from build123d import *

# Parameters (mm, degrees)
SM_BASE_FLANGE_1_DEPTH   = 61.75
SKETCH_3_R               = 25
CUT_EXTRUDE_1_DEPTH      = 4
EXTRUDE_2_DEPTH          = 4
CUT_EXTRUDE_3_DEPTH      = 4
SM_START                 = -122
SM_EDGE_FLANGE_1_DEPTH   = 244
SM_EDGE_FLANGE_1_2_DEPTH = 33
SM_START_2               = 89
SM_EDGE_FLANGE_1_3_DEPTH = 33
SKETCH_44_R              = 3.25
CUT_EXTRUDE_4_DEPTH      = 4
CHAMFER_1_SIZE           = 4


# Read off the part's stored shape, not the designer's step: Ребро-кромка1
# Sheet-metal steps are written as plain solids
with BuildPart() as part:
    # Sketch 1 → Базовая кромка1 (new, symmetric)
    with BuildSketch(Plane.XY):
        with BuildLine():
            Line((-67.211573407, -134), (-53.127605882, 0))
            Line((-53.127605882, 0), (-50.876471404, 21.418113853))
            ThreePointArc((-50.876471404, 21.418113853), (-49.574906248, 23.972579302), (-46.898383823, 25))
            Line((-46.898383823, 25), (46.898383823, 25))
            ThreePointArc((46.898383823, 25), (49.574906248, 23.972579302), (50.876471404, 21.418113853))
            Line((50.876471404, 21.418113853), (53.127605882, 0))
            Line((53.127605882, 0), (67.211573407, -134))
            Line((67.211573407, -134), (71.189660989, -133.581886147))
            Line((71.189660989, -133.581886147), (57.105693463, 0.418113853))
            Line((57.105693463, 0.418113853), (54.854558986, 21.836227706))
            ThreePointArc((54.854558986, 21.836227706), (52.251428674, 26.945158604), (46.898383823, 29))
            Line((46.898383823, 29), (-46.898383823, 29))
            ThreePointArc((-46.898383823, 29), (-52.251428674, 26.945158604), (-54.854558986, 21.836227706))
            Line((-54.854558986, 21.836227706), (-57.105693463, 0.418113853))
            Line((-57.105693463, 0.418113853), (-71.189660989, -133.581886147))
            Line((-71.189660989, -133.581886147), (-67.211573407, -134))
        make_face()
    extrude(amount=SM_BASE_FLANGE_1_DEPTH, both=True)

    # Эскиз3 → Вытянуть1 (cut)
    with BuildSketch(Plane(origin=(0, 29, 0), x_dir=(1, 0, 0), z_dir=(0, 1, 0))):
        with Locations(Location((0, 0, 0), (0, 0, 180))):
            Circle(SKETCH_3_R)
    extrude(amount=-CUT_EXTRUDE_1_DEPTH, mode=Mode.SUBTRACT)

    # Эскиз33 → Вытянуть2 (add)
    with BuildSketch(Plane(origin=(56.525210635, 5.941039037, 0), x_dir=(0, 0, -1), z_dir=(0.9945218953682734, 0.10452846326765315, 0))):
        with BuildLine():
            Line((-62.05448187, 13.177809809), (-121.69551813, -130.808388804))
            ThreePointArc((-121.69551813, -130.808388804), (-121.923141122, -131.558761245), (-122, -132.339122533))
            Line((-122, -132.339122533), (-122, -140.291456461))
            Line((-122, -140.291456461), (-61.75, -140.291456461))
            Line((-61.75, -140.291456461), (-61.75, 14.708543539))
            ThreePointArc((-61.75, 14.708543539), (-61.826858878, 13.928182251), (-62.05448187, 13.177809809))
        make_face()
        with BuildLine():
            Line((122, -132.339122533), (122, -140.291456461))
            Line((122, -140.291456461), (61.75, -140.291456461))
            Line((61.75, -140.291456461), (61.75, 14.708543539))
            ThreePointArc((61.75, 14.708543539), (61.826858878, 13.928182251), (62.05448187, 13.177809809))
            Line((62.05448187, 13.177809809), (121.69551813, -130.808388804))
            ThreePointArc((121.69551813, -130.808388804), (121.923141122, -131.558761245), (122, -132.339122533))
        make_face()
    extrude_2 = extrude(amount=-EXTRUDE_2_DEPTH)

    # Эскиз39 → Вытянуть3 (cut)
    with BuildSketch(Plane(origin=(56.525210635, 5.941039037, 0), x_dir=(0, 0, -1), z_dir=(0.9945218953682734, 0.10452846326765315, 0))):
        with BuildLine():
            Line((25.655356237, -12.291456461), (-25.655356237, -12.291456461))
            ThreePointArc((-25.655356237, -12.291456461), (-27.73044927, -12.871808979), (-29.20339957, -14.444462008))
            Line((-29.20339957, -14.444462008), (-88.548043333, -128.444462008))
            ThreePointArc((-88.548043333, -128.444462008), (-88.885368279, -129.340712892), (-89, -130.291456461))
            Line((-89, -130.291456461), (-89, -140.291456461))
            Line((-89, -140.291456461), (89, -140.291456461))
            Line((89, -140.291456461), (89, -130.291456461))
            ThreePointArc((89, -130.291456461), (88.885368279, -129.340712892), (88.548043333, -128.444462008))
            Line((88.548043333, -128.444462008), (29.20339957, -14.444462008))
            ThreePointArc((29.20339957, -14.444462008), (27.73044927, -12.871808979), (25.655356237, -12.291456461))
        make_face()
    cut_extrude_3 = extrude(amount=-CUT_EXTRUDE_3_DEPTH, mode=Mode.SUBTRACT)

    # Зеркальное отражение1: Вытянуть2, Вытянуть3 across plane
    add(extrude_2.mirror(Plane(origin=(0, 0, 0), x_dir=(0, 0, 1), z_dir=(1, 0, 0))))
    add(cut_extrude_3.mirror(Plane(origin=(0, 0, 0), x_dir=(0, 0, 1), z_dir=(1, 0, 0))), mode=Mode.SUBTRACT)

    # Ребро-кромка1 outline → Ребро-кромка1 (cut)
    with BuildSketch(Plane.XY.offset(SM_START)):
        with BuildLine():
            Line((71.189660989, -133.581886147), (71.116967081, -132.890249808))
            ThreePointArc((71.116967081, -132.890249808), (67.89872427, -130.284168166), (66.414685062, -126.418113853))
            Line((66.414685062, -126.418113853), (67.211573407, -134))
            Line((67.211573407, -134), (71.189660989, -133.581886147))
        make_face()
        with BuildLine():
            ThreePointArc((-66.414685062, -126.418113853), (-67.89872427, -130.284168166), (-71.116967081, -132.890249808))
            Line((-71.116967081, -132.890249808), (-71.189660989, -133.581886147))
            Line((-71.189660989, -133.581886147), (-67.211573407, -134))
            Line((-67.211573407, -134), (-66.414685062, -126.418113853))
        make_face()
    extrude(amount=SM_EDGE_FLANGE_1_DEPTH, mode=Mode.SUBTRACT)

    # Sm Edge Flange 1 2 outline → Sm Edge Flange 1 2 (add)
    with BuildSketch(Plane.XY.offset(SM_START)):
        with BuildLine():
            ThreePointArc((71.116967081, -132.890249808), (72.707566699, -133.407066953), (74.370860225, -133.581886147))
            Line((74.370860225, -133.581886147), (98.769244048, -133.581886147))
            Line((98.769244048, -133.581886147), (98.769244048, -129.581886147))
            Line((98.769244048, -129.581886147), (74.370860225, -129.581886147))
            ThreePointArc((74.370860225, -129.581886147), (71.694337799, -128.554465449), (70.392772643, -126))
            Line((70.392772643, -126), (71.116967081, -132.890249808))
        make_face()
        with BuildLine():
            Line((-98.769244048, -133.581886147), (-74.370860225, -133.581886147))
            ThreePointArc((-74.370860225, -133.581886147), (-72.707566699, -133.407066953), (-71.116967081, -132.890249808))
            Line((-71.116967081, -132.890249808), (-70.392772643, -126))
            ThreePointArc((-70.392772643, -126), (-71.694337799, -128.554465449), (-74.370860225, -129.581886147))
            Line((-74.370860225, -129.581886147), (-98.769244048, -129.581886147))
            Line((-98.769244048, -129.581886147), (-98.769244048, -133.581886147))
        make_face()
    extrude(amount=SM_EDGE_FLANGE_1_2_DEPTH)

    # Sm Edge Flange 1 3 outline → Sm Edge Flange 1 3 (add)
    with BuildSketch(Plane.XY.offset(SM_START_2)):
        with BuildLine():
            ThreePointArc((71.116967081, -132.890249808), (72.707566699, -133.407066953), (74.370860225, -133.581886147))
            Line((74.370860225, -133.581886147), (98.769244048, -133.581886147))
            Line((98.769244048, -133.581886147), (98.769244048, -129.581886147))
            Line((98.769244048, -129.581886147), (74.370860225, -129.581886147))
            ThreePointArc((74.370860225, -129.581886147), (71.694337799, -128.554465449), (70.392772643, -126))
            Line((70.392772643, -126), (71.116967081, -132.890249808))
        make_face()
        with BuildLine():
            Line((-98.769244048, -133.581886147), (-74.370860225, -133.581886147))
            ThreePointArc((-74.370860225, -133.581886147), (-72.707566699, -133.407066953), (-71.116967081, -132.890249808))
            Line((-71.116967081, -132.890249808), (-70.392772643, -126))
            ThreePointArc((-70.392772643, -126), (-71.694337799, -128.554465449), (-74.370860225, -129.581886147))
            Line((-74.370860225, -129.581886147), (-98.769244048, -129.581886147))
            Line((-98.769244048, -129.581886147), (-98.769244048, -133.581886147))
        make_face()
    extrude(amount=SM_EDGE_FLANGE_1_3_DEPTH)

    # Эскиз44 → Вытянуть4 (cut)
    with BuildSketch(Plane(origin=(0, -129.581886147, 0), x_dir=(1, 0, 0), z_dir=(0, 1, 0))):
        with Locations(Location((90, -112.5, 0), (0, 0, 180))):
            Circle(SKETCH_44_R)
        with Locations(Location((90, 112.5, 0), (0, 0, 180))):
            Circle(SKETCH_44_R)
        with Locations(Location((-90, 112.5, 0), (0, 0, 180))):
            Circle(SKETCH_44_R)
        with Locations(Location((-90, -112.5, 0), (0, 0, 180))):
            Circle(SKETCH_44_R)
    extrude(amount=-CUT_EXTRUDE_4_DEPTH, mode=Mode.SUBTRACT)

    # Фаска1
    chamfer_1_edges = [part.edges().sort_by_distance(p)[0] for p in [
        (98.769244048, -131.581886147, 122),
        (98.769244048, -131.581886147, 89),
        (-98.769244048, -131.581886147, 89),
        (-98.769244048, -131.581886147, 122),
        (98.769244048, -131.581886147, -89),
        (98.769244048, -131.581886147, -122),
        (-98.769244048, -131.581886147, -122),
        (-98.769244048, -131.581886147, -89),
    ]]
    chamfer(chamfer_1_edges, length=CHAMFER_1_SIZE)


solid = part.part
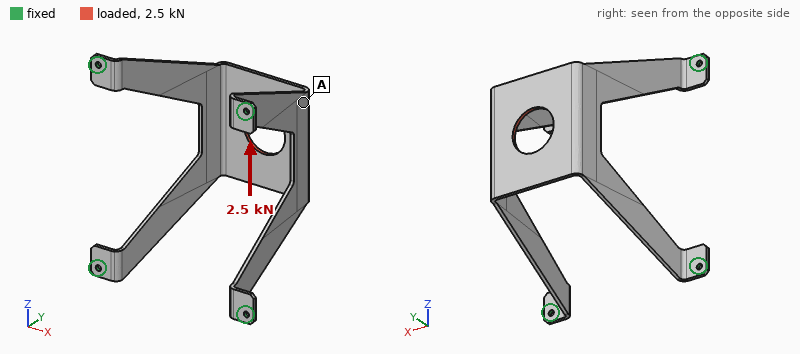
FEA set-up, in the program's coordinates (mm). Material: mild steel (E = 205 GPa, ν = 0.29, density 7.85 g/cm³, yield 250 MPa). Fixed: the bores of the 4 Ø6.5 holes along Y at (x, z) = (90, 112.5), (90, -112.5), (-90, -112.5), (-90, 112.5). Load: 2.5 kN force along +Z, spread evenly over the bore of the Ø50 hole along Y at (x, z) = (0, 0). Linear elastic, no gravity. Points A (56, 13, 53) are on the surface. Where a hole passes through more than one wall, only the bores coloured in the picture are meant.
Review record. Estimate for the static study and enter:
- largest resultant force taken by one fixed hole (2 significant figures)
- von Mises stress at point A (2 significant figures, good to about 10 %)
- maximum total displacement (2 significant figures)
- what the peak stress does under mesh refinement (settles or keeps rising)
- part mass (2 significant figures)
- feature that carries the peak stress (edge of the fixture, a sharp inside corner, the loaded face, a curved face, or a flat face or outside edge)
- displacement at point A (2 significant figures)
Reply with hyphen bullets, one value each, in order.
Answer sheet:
- 1.1 kN
- 17 MPa
- 0.14 mm
- keeps rising
- 1.3 kg
- edge of the fixture
- 0.12 mm
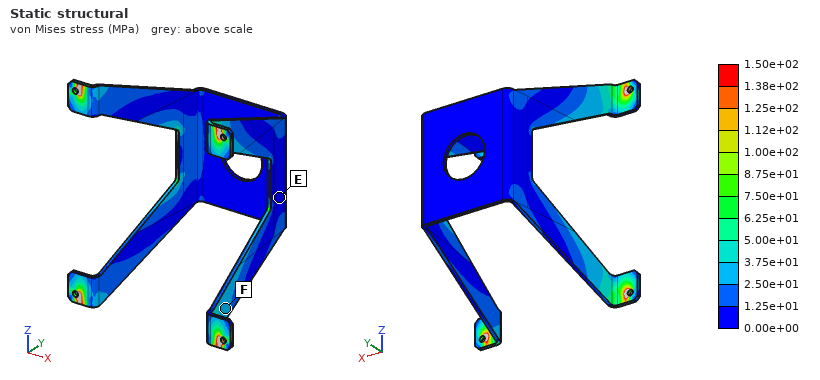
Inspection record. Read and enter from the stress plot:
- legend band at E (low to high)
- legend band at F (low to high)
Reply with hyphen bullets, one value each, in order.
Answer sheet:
- 0.00e+00 to 1.25e+01 MPa
- 2.50e+01 to 3.75e+01 MPa
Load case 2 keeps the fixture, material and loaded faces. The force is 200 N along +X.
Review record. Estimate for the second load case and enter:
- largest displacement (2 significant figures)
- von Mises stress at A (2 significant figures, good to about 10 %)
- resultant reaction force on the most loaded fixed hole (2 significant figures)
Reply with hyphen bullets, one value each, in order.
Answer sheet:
- 0.47 mm
- 26 MPa
- 95 N
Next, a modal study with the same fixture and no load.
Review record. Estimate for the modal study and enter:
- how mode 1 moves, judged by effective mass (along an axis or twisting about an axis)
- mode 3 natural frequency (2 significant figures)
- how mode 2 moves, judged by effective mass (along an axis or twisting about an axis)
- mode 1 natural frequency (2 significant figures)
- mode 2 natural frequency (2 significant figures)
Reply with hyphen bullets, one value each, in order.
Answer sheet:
- along X
- 490 Hz
- twisting about Y
- 120 Hz
- 450 Hz
